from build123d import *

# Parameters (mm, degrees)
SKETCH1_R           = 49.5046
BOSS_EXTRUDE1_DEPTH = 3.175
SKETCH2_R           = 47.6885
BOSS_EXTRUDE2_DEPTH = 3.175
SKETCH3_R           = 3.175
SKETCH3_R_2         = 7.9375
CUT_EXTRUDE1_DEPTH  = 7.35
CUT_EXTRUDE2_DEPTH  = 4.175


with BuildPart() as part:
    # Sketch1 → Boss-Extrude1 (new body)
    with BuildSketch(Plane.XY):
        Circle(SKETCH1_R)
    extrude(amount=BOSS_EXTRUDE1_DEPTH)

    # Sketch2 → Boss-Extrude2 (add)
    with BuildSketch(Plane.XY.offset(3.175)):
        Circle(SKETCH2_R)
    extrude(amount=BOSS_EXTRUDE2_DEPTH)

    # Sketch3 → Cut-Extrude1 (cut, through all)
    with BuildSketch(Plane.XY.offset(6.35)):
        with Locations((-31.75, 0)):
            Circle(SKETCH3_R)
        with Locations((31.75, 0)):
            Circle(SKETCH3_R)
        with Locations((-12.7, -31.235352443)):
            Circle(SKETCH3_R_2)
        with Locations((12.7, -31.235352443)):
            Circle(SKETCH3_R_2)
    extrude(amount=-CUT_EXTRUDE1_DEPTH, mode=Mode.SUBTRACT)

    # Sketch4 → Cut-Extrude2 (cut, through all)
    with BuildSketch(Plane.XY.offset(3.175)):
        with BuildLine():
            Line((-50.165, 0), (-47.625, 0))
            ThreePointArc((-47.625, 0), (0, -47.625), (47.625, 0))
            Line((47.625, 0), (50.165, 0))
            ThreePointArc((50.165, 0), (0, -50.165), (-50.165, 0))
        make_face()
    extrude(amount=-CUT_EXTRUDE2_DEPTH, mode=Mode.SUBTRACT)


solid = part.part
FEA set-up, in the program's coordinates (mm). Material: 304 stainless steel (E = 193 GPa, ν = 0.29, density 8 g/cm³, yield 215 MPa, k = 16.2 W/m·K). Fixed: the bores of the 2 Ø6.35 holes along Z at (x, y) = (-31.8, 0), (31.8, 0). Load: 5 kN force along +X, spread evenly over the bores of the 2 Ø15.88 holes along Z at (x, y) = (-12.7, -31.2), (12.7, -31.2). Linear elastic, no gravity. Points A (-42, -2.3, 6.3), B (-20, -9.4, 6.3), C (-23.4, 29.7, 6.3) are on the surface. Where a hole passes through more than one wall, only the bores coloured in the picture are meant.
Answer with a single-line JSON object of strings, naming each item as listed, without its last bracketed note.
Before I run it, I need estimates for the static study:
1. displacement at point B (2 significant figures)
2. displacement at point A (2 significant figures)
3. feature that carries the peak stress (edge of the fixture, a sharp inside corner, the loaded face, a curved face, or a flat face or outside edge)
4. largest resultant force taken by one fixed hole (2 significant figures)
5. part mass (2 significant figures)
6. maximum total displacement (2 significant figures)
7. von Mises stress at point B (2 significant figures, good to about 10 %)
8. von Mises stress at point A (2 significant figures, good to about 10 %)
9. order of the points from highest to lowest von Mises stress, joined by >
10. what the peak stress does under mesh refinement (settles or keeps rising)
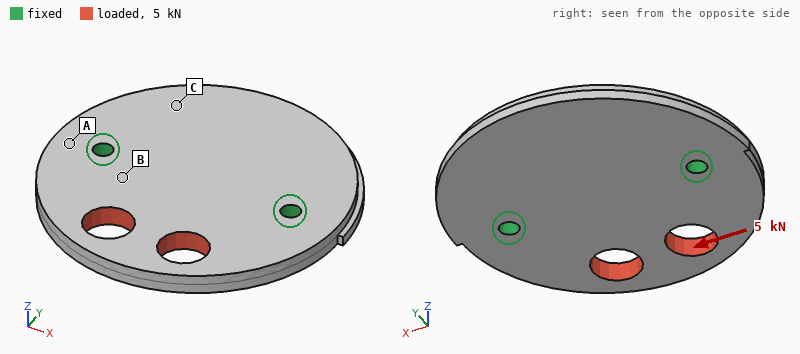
{"displacement at point B": "1.9 µm", "displacement at point A": "1.6 µm", "feature that carries the peak stress": "edge of the fixture", "largest resultant force taken by one fixed hole": "3.4 kN", "part mass": "350 g", "maximum total displacement": "9.9 µm", "von Mises stress at point B": "22 MPa", "von Mises stress at point A": "12 MPa", "order of the points from highest to lowest von Mises stress, joined by >": "B > A > C", "what the peak stress does under mesh refinement": "keeps rising"}
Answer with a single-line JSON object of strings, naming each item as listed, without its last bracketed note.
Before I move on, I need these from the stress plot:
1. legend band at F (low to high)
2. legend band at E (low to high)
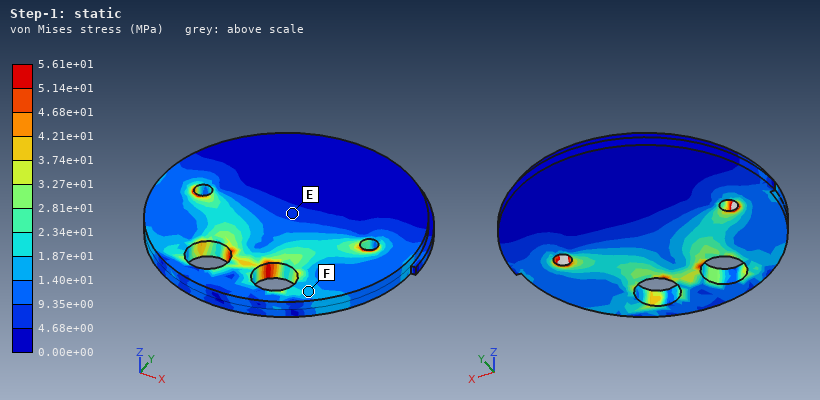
{"legend band at F": "1.40e+01 to 1.87e+01 MPa", "legend band at E": "4.68e+00 to 9.35e+00 MPa"}
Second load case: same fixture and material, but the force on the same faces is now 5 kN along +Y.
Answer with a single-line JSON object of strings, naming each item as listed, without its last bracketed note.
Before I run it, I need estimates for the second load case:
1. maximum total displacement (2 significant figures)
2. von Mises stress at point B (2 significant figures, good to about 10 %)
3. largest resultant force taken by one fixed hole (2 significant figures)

{"maximum total displacement": "4.8 µm", "von Mises stress at point B": "13 MPa", "largest resultant force taken by one fixed hole": "2.5 kN"}
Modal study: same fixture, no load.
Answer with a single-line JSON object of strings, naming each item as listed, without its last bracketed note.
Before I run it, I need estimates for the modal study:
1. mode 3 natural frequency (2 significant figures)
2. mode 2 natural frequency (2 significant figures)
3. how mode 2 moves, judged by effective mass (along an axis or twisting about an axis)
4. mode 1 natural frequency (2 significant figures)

{"mode 3 natural frequency": "5300 Hz", "mode 2 natural frequency": "2900 Hz", "how mode 2 moves, judged by effective mass": "along Z", "mode 1 natural frequency": "2200 Hz"}
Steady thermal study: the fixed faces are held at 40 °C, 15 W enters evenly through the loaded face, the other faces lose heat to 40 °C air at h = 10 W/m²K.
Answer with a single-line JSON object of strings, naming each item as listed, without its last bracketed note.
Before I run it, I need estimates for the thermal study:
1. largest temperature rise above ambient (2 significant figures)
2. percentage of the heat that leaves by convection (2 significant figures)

{"largest temperature rise above ambient": "86 K", "percentage of the heat that leaves by convection": "24 %"}
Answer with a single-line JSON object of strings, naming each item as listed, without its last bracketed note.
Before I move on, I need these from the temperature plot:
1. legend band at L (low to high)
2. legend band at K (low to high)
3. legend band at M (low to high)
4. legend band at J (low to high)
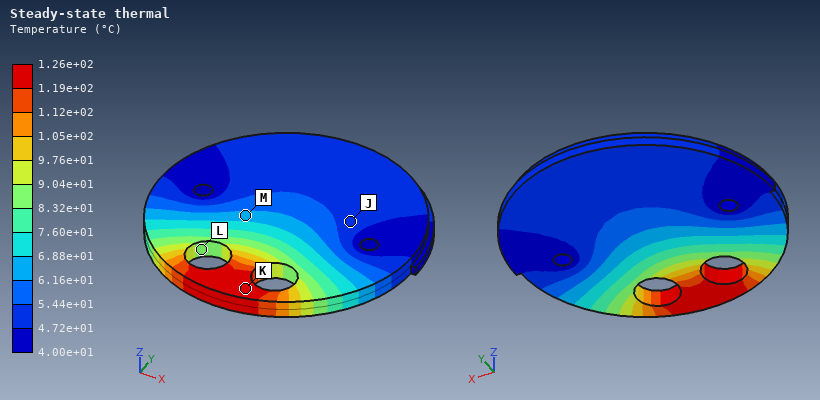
{"legend band at L": "8.32e+01 to 9.04e+01 °C", "legend band at K": "1.19e+02 to 1.26e+02 °C", "legend band at M": "6.16e+01 to 6.88e+01 °C", "legend band at J": "4.72e+01 to 5.44e+01 °C"}
